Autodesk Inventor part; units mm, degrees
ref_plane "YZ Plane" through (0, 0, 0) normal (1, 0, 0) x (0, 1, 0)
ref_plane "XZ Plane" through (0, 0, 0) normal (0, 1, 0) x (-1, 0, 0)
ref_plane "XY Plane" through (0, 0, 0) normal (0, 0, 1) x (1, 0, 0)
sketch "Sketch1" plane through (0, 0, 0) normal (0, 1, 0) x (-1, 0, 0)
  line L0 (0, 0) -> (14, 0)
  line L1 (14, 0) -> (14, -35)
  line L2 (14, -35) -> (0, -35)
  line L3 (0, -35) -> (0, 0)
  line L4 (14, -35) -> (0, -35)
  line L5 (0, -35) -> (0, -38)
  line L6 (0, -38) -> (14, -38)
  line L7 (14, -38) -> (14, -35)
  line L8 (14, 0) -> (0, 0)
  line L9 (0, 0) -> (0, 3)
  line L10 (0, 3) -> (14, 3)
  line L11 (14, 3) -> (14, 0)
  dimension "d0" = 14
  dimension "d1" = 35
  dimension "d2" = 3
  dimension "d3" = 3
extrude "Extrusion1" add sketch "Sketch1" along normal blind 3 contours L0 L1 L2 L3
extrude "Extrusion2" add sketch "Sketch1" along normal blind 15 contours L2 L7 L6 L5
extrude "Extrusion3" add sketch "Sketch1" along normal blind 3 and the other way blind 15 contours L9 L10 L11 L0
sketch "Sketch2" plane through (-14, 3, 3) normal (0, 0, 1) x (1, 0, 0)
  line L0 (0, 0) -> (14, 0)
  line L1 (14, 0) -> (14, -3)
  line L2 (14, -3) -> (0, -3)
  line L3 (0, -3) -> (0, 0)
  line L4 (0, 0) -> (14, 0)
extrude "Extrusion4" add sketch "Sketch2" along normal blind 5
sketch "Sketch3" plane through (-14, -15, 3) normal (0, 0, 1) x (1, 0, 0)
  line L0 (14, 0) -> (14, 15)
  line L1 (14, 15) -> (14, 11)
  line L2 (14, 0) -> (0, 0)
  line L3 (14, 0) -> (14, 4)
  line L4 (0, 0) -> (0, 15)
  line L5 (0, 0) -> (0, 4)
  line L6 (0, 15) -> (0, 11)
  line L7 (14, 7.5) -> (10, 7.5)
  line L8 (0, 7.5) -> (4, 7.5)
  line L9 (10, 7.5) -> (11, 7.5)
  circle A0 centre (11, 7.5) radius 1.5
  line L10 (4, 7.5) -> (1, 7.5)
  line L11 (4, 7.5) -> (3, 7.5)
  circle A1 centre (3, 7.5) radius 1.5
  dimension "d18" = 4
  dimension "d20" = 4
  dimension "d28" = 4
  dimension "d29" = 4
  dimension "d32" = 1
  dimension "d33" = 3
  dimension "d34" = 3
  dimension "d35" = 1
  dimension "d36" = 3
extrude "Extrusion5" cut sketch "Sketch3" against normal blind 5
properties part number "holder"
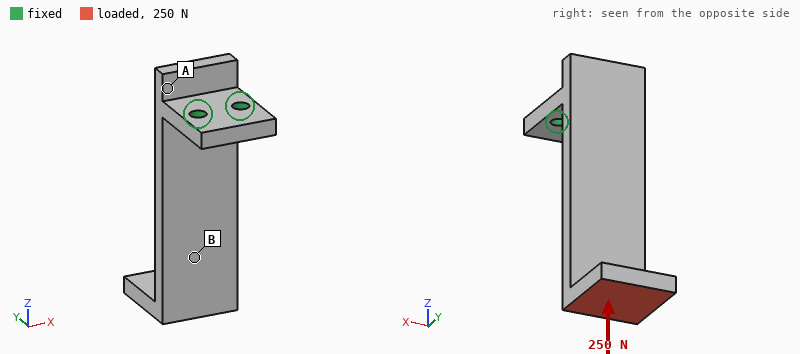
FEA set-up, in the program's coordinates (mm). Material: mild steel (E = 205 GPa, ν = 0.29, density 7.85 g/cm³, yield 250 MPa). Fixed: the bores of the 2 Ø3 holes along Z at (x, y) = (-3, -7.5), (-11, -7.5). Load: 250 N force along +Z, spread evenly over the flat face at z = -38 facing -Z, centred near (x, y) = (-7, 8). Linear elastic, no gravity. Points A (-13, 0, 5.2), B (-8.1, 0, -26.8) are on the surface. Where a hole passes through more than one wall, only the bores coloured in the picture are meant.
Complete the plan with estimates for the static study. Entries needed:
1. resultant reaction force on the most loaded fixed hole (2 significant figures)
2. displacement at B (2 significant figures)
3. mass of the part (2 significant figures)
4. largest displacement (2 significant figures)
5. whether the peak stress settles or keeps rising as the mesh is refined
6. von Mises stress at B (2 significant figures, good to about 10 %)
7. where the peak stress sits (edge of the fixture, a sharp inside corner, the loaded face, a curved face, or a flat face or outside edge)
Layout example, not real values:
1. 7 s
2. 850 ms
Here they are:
1. 130 N
2. 0.17 mm
3. 24 g
4. 0.34 mm
5. keeps rising
6. 63 MPa
7. edge of the fixture
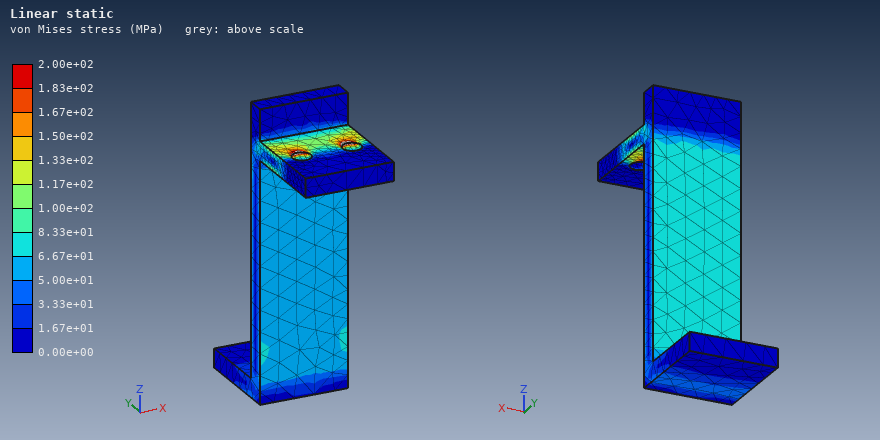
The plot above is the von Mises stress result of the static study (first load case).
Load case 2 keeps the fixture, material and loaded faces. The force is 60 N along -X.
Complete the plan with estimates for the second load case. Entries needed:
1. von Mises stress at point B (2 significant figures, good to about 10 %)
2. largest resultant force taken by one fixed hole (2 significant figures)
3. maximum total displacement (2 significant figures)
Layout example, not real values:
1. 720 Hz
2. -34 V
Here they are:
1. 13 MPa
2. 250 N
3. 61 µm
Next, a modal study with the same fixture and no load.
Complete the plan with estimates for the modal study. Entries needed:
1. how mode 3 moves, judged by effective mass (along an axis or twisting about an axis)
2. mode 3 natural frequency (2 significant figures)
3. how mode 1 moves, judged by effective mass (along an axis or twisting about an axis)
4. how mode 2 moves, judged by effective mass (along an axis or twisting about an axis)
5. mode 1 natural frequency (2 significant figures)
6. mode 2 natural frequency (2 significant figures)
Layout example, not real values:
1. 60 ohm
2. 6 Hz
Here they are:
1. twisting about Z
2. 4600 Hz
3. along Y
4. along X
5. 840 Hz
6. 2000 Hz
